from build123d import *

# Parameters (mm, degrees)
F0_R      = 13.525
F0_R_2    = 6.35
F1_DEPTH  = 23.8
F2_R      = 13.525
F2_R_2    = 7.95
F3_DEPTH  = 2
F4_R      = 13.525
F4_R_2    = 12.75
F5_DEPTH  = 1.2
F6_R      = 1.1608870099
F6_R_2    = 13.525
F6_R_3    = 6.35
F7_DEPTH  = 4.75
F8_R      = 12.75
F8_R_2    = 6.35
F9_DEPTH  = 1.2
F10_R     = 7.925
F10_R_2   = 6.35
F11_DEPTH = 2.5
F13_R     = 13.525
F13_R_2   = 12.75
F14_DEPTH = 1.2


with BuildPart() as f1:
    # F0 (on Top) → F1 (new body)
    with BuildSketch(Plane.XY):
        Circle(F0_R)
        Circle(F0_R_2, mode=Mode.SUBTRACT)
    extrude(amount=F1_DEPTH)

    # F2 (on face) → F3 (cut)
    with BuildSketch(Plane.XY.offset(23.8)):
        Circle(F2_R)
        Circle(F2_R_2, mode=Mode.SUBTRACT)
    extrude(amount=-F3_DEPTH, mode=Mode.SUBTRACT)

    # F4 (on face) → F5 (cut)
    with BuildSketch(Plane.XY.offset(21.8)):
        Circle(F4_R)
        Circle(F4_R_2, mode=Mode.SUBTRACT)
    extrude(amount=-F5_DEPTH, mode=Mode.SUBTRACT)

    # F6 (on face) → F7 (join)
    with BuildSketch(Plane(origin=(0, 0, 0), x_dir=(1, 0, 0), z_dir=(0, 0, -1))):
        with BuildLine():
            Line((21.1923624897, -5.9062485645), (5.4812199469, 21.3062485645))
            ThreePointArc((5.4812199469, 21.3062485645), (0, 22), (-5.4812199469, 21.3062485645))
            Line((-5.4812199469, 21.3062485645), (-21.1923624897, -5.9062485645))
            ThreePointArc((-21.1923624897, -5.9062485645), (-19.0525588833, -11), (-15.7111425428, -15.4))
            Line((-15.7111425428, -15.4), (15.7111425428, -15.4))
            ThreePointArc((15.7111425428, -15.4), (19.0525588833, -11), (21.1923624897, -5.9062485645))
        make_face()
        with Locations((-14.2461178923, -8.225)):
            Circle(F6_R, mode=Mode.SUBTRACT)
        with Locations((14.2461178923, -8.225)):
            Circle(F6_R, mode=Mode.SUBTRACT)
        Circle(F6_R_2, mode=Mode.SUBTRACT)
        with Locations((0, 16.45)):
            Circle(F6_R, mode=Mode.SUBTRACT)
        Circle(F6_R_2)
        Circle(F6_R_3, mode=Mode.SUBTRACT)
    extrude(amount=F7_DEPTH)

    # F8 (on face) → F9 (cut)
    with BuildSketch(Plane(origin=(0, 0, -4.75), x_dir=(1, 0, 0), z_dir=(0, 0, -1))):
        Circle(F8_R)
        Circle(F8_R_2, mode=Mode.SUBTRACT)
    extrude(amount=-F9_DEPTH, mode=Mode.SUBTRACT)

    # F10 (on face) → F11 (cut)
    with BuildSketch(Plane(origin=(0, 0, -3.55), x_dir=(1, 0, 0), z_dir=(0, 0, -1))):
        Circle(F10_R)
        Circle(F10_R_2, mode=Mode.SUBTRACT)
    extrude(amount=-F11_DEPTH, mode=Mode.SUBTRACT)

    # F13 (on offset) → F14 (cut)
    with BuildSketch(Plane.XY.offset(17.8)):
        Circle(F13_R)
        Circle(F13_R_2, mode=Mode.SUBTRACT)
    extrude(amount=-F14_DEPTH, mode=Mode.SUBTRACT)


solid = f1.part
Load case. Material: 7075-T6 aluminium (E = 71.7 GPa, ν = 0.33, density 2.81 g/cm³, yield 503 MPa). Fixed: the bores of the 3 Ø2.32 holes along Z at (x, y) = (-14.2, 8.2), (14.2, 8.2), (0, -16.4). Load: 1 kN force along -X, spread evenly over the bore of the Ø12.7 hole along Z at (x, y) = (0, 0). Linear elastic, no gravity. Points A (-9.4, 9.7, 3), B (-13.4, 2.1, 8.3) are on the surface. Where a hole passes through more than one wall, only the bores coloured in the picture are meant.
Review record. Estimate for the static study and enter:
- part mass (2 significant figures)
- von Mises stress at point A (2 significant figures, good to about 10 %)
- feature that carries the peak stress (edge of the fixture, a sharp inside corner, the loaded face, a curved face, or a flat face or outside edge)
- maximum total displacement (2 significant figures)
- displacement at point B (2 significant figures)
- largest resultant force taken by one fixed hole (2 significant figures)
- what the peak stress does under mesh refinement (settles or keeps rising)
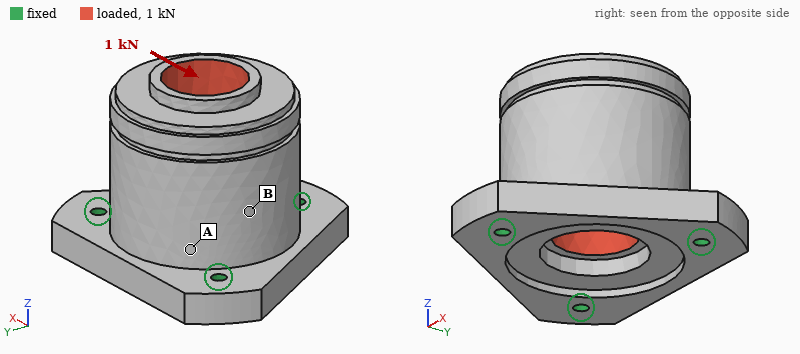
38 g
13 MPa
edge of the fixture
11 µm
5.9 µm
640 N
keeps rising
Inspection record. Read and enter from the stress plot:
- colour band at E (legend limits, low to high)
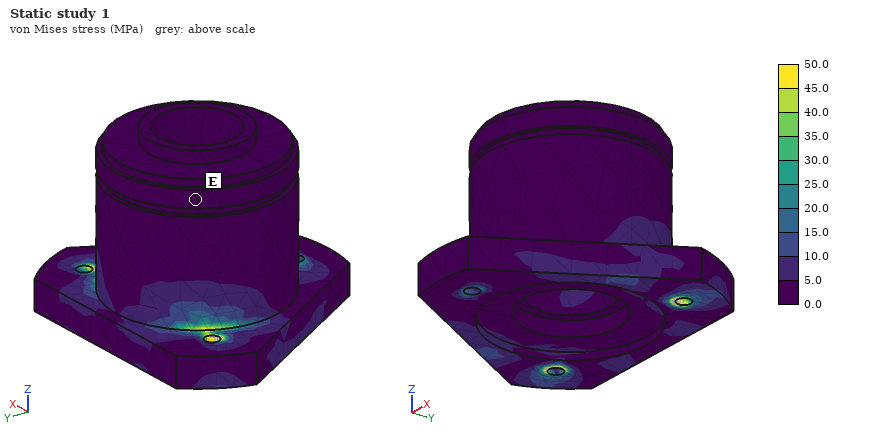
0.0 to 5.0 MPa
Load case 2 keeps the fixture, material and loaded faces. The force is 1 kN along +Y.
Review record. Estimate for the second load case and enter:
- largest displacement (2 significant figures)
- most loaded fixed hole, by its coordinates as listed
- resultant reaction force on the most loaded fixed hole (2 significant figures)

11 µm
(0, -16.4)
730 N
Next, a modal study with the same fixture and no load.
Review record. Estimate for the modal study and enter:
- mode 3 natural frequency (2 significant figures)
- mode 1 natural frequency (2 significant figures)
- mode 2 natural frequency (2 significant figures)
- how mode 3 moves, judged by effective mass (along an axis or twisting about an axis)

17 kHz
11 kHz
11 kHz
along Z
